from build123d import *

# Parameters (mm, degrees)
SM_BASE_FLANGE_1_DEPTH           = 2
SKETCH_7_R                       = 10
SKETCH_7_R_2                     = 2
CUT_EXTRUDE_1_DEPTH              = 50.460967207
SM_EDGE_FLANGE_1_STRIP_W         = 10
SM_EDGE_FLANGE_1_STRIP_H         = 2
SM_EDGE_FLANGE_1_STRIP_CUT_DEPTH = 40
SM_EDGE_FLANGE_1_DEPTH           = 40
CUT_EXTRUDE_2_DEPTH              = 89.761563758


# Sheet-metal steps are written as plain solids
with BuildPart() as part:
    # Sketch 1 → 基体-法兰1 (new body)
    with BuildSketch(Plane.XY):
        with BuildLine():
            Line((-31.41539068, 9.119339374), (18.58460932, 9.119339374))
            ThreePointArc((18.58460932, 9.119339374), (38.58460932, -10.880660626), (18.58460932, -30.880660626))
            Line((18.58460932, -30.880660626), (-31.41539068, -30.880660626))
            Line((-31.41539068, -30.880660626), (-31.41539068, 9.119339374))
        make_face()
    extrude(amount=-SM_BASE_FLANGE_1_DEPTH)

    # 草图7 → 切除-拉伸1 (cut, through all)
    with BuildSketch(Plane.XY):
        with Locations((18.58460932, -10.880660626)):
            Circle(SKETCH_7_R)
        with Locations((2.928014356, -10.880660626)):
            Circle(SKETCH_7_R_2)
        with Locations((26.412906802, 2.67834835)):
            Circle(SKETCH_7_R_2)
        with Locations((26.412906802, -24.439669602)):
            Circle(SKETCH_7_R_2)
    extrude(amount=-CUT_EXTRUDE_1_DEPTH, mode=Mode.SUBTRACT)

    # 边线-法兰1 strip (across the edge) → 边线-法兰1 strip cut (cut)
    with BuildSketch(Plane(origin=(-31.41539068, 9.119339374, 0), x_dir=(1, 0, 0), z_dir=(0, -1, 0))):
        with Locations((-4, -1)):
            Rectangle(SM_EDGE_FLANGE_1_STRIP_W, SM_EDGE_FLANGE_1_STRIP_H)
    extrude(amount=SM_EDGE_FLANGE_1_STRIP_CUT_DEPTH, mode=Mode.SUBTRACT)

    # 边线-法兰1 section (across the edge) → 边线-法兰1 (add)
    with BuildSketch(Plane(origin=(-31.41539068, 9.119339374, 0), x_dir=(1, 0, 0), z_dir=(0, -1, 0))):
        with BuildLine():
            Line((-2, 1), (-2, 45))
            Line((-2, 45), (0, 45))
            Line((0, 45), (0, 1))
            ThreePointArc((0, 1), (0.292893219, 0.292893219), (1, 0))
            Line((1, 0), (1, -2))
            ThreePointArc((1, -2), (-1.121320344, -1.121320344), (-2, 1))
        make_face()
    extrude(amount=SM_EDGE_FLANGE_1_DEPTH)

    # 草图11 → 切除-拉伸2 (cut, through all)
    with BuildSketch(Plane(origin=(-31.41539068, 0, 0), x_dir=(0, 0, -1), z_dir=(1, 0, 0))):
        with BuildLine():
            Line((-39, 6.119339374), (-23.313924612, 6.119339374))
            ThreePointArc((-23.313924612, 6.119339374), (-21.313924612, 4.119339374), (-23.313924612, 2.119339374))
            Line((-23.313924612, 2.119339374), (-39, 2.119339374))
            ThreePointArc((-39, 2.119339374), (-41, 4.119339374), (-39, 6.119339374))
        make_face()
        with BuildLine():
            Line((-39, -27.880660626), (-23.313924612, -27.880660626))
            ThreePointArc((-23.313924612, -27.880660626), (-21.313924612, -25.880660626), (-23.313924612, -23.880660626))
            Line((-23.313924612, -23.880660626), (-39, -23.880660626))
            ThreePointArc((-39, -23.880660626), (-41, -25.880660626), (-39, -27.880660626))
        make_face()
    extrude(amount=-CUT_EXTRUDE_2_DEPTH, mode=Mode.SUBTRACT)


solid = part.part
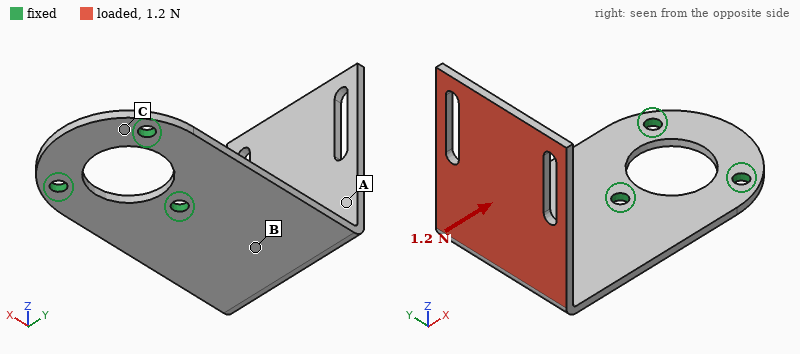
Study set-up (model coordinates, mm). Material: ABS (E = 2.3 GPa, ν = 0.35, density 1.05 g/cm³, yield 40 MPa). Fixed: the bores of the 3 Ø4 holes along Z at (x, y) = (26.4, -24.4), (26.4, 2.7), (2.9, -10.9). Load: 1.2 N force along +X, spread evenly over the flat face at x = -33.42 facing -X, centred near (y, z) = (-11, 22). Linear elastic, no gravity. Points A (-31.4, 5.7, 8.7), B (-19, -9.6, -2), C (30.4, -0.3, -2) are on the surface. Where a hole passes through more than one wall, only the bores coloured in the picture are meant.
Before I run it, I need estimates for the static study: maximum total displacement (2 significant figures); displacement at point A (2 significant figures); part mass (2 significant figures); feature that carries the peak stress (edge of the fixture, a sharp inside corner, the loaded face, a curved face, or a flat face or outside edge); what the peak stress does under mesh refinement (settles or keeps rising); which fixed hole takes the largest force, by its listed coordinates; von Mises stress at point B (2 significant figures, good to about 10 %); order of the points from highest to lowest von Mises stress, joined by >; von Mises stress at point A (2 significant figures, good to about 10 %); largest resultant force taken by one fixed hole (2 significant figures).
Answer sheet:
0.96 mm
0.31 mm
8.3 g
edge of the fixture
keeps rising
(2.9, -10.9)
0.89 MPa
B > A > C
0.58 MPa
1.0 N
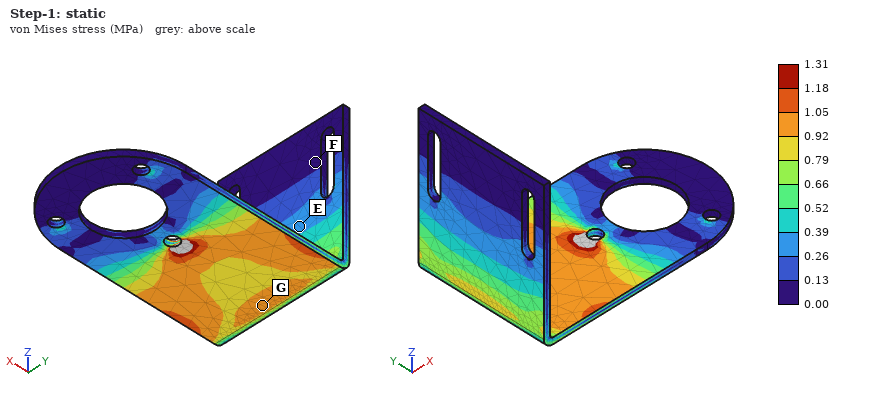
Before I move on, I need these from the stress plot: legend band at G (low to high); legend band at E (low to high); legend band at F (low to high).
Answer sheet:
0.92 to 1.05 MPa
0.26 to 0.39 MPa
0.00 to 0.13 MPa
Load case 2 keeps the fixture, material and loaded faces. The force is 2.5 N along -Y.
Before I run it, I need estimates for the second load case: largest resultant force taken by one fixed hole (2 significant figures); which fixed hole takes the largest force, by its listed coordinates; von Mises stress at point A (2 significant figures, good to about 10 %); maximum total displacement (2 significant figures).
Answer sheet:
3.3 N
(2.9, -10.9)
0.66 MPa
1.1 mm
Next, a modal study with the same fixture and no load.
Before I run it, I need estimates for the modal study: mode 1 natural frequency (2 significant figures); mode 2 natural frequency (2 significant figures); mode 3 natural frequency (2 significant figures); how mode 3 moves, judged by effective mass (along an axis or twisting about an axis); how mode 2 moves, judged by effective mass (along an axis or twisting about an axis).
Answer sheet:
100 Hz
150 Hz
280 Hz
along Z
along Y
